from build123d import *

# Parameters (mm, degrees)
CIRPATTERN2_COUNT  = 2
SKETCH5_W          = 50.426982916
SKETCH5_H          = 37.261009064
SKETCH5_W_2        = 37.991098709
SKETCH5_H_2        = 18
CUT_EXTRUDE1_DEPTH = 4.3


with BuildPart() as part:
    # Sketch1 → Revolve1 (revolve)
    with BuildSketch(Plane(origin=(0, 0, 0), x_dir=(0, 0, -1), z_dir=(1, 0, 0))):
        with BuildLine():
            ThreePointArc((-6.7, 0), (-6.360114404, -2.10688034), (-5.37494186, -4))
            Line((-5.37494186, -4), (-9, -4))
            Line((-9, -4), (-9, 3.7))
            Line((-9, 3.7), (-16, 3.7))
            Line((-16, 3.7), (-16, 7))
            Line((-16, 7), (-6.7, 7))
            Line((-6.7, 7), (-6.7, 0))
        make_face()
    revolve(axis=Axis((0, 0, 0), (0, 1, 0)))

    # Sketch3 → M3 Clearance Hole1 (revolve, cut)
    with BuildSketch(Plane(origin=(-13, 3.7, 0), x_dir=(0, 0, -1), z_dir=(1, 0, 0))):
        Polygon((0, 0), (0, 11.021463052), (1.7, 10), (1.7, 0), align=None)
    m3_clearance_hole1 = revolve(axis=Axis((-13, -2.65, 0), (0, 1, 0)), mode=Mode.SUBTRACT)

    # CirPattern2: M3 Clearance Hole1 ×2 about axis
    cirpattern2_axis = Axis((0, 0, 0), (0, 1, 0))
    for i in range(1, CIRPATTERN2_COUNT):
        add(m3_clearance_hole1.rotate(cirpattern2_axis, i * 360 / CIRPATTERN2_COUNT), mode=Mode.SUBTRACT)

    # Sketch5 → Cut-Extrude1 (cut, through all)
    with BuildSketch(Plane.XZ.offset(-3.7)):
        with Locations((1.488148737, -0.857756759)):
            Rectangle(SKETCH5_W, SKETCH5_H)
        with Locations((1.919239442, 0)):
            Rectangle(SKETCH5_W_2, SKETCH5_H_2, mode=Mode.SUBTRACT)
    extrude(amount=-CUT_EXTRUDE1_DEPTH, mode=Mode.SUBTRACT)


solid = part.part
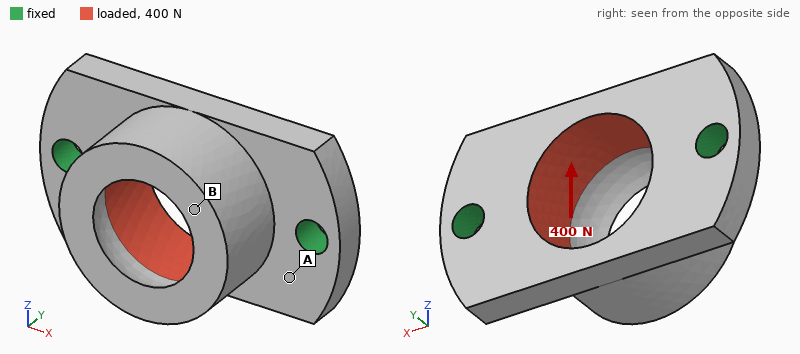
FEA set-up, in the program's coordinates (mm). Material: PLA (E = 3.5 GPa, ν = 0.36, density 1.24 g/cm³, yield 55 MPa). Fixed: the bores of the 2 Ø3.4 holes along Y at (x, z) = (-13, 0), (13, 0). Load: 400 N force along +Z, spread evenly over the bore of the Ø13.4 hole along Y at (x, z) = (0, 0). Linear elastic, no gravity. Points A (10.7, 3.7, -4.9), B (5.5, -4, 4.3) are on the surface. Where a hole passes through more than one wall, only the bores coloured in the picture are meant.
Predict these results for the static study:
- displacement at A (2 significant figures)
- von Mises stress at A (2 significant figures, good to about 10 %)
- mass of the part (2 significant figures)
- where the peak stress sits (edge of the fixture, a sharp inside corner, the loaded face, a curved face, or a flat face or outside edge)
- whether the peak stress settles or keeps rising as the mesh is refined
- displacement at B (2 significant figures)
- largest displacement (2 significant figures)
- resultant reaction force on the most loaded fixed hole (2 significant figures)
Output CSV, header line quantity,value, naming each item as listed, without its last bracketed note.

quantity,value
displacement at A,0.031 mm
von Mises stress at A,8.8 MPa
mass of the part,2.7 g
where the peak stress sits,edge of the fixture
whether the peak stress settles or keeps rising as the mesh is refined,keeps rising
displacement at B,0.12 mm
largest displacement,0.14 mm
resultant reaction force on the most loaded fixed hole,200 N
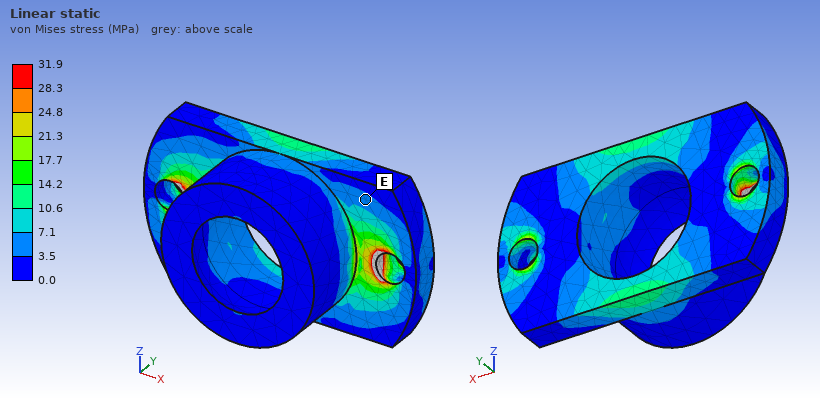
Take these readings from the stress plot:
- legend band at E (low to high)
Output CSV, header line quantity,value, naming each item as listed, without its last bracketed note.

quantity,value
legend band at E,3.5 to 7.1 MPa
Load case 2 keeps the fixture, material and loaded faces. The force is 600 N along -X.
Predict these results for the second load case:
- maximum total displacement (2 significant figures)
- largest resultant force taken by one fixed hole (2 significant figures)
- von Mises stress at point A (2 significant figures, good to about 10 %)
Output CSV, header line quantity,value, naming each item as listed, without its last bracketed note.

quantity,value
maximum total displacement,38 µm
largest resultant force taken by one fixed hole,300 N
von Mises stress at point A,6.6 MPa
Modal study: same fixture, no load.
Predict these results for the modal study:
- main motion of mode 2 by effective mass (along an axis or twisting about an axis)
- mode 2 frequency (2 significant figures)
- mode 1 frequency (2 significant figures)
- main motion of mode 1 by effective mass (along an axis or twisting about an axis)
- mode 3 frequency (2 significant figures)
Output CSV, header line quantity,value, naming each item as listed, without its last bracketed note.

quantity,value
main motion of mode 2 by effective mass,along Y
mode 2 frequency,7500 Hz
mode 1 frequency,4200 Hz
main motion of mode 1 by effective mass,along Z
mode 3 frequency,11 kHz
